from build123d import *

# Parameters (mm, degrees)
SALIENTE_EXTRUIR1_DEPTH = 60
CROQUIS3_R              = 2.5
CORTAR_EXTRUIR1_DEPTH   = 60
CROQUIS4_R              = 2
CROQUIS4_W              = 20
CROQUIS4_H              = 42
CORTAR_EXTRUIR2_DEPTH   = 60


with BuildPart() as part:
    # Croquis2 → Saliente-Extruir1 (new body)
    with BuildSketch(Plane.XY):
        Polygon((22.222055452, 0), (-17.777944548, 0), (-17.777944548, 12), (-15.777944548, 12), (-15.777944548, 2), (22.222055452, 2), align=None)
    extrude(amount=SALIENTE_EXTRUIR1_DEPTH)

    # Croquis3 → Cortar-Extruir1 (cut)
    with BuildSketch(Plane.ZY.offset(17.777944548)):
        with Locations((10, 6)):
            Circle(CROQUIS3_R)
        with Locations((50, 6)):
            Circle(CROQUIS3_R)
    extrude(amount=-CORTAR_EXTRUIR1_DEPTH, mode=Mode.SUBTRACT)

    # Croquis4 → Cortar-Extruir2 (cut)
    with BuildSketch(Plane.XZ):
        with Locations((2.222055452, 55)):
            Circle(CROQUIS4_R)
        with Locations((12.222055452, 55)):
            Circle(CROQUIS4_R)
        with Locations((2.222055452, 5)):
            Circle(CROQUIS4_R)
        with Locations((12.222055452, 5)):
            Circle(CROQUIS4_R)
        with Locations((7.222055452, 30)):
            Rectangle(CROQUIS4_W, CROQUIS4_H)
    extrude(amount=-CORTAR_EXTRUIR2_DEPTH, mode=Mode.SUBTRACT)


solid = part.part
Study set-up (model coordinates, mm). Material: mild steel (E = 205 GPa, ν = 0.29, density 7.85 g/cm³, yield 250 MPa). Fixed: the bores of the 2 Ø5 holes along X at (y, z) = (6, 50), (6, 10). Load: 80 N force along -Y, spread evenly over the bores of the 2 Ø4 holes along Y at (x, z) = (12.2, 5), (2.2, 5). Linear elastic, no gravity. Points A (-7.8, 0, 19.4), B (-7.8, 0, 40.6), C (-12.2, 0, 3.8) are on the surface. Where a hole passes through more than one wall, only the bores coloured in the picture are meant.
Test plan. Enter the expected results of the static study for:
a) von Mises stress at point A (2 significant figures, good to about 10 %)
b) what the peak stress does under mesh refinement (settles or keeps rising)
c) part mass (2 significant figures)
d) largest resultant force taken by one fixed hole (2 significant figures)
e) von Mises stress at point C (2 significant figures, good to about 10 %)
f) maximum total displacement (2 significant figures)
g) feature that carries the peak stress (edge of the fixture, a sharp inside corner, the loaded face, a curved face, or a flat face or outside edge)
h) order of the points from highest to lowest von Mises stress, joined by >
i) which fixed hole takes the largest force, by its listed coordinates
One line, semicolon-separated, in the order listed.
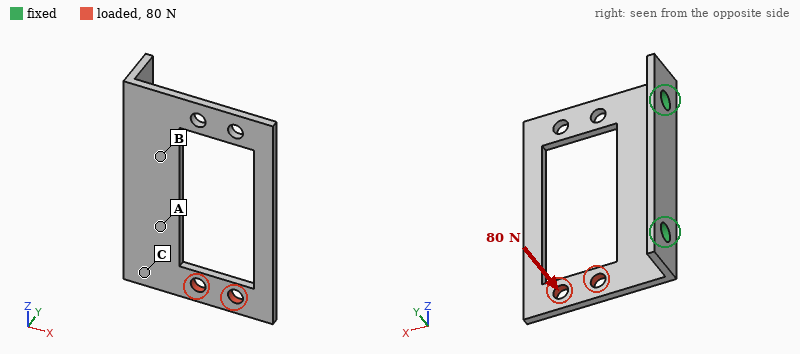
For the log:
52 MPa; keeps rising; 33 g; 83 N; 96 MPa; 0.36 mm; edge of the fixture; C > A > B; (6, 10)
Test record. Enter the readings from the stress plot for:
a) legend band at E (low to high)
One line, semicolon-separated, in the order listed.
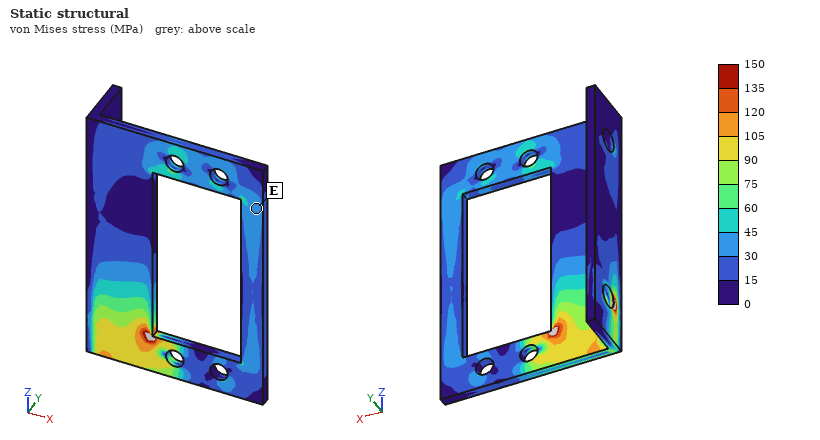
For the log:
30 to 45 MPa
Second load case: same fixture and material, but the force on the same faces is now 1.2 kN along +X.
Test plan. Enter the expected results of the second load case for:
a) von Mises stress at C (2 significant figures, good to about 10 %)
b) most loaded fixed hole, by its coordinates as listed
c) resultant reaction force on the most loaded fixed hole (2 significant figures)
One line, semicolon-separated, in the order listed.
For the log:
54 MPa; (6, 10); 1.3 kN
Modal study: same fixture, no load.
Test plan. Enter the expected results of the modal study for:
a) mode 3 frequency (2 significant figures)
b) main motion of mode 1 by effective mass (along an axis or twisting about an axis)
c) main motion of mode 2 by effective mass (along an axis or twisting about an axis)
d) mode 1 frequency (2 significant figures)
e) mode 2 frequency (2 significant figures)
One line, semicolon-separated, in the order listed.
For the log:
3300 Hz; along Y; twisting about X; 860 Hz; 1500 Hz
